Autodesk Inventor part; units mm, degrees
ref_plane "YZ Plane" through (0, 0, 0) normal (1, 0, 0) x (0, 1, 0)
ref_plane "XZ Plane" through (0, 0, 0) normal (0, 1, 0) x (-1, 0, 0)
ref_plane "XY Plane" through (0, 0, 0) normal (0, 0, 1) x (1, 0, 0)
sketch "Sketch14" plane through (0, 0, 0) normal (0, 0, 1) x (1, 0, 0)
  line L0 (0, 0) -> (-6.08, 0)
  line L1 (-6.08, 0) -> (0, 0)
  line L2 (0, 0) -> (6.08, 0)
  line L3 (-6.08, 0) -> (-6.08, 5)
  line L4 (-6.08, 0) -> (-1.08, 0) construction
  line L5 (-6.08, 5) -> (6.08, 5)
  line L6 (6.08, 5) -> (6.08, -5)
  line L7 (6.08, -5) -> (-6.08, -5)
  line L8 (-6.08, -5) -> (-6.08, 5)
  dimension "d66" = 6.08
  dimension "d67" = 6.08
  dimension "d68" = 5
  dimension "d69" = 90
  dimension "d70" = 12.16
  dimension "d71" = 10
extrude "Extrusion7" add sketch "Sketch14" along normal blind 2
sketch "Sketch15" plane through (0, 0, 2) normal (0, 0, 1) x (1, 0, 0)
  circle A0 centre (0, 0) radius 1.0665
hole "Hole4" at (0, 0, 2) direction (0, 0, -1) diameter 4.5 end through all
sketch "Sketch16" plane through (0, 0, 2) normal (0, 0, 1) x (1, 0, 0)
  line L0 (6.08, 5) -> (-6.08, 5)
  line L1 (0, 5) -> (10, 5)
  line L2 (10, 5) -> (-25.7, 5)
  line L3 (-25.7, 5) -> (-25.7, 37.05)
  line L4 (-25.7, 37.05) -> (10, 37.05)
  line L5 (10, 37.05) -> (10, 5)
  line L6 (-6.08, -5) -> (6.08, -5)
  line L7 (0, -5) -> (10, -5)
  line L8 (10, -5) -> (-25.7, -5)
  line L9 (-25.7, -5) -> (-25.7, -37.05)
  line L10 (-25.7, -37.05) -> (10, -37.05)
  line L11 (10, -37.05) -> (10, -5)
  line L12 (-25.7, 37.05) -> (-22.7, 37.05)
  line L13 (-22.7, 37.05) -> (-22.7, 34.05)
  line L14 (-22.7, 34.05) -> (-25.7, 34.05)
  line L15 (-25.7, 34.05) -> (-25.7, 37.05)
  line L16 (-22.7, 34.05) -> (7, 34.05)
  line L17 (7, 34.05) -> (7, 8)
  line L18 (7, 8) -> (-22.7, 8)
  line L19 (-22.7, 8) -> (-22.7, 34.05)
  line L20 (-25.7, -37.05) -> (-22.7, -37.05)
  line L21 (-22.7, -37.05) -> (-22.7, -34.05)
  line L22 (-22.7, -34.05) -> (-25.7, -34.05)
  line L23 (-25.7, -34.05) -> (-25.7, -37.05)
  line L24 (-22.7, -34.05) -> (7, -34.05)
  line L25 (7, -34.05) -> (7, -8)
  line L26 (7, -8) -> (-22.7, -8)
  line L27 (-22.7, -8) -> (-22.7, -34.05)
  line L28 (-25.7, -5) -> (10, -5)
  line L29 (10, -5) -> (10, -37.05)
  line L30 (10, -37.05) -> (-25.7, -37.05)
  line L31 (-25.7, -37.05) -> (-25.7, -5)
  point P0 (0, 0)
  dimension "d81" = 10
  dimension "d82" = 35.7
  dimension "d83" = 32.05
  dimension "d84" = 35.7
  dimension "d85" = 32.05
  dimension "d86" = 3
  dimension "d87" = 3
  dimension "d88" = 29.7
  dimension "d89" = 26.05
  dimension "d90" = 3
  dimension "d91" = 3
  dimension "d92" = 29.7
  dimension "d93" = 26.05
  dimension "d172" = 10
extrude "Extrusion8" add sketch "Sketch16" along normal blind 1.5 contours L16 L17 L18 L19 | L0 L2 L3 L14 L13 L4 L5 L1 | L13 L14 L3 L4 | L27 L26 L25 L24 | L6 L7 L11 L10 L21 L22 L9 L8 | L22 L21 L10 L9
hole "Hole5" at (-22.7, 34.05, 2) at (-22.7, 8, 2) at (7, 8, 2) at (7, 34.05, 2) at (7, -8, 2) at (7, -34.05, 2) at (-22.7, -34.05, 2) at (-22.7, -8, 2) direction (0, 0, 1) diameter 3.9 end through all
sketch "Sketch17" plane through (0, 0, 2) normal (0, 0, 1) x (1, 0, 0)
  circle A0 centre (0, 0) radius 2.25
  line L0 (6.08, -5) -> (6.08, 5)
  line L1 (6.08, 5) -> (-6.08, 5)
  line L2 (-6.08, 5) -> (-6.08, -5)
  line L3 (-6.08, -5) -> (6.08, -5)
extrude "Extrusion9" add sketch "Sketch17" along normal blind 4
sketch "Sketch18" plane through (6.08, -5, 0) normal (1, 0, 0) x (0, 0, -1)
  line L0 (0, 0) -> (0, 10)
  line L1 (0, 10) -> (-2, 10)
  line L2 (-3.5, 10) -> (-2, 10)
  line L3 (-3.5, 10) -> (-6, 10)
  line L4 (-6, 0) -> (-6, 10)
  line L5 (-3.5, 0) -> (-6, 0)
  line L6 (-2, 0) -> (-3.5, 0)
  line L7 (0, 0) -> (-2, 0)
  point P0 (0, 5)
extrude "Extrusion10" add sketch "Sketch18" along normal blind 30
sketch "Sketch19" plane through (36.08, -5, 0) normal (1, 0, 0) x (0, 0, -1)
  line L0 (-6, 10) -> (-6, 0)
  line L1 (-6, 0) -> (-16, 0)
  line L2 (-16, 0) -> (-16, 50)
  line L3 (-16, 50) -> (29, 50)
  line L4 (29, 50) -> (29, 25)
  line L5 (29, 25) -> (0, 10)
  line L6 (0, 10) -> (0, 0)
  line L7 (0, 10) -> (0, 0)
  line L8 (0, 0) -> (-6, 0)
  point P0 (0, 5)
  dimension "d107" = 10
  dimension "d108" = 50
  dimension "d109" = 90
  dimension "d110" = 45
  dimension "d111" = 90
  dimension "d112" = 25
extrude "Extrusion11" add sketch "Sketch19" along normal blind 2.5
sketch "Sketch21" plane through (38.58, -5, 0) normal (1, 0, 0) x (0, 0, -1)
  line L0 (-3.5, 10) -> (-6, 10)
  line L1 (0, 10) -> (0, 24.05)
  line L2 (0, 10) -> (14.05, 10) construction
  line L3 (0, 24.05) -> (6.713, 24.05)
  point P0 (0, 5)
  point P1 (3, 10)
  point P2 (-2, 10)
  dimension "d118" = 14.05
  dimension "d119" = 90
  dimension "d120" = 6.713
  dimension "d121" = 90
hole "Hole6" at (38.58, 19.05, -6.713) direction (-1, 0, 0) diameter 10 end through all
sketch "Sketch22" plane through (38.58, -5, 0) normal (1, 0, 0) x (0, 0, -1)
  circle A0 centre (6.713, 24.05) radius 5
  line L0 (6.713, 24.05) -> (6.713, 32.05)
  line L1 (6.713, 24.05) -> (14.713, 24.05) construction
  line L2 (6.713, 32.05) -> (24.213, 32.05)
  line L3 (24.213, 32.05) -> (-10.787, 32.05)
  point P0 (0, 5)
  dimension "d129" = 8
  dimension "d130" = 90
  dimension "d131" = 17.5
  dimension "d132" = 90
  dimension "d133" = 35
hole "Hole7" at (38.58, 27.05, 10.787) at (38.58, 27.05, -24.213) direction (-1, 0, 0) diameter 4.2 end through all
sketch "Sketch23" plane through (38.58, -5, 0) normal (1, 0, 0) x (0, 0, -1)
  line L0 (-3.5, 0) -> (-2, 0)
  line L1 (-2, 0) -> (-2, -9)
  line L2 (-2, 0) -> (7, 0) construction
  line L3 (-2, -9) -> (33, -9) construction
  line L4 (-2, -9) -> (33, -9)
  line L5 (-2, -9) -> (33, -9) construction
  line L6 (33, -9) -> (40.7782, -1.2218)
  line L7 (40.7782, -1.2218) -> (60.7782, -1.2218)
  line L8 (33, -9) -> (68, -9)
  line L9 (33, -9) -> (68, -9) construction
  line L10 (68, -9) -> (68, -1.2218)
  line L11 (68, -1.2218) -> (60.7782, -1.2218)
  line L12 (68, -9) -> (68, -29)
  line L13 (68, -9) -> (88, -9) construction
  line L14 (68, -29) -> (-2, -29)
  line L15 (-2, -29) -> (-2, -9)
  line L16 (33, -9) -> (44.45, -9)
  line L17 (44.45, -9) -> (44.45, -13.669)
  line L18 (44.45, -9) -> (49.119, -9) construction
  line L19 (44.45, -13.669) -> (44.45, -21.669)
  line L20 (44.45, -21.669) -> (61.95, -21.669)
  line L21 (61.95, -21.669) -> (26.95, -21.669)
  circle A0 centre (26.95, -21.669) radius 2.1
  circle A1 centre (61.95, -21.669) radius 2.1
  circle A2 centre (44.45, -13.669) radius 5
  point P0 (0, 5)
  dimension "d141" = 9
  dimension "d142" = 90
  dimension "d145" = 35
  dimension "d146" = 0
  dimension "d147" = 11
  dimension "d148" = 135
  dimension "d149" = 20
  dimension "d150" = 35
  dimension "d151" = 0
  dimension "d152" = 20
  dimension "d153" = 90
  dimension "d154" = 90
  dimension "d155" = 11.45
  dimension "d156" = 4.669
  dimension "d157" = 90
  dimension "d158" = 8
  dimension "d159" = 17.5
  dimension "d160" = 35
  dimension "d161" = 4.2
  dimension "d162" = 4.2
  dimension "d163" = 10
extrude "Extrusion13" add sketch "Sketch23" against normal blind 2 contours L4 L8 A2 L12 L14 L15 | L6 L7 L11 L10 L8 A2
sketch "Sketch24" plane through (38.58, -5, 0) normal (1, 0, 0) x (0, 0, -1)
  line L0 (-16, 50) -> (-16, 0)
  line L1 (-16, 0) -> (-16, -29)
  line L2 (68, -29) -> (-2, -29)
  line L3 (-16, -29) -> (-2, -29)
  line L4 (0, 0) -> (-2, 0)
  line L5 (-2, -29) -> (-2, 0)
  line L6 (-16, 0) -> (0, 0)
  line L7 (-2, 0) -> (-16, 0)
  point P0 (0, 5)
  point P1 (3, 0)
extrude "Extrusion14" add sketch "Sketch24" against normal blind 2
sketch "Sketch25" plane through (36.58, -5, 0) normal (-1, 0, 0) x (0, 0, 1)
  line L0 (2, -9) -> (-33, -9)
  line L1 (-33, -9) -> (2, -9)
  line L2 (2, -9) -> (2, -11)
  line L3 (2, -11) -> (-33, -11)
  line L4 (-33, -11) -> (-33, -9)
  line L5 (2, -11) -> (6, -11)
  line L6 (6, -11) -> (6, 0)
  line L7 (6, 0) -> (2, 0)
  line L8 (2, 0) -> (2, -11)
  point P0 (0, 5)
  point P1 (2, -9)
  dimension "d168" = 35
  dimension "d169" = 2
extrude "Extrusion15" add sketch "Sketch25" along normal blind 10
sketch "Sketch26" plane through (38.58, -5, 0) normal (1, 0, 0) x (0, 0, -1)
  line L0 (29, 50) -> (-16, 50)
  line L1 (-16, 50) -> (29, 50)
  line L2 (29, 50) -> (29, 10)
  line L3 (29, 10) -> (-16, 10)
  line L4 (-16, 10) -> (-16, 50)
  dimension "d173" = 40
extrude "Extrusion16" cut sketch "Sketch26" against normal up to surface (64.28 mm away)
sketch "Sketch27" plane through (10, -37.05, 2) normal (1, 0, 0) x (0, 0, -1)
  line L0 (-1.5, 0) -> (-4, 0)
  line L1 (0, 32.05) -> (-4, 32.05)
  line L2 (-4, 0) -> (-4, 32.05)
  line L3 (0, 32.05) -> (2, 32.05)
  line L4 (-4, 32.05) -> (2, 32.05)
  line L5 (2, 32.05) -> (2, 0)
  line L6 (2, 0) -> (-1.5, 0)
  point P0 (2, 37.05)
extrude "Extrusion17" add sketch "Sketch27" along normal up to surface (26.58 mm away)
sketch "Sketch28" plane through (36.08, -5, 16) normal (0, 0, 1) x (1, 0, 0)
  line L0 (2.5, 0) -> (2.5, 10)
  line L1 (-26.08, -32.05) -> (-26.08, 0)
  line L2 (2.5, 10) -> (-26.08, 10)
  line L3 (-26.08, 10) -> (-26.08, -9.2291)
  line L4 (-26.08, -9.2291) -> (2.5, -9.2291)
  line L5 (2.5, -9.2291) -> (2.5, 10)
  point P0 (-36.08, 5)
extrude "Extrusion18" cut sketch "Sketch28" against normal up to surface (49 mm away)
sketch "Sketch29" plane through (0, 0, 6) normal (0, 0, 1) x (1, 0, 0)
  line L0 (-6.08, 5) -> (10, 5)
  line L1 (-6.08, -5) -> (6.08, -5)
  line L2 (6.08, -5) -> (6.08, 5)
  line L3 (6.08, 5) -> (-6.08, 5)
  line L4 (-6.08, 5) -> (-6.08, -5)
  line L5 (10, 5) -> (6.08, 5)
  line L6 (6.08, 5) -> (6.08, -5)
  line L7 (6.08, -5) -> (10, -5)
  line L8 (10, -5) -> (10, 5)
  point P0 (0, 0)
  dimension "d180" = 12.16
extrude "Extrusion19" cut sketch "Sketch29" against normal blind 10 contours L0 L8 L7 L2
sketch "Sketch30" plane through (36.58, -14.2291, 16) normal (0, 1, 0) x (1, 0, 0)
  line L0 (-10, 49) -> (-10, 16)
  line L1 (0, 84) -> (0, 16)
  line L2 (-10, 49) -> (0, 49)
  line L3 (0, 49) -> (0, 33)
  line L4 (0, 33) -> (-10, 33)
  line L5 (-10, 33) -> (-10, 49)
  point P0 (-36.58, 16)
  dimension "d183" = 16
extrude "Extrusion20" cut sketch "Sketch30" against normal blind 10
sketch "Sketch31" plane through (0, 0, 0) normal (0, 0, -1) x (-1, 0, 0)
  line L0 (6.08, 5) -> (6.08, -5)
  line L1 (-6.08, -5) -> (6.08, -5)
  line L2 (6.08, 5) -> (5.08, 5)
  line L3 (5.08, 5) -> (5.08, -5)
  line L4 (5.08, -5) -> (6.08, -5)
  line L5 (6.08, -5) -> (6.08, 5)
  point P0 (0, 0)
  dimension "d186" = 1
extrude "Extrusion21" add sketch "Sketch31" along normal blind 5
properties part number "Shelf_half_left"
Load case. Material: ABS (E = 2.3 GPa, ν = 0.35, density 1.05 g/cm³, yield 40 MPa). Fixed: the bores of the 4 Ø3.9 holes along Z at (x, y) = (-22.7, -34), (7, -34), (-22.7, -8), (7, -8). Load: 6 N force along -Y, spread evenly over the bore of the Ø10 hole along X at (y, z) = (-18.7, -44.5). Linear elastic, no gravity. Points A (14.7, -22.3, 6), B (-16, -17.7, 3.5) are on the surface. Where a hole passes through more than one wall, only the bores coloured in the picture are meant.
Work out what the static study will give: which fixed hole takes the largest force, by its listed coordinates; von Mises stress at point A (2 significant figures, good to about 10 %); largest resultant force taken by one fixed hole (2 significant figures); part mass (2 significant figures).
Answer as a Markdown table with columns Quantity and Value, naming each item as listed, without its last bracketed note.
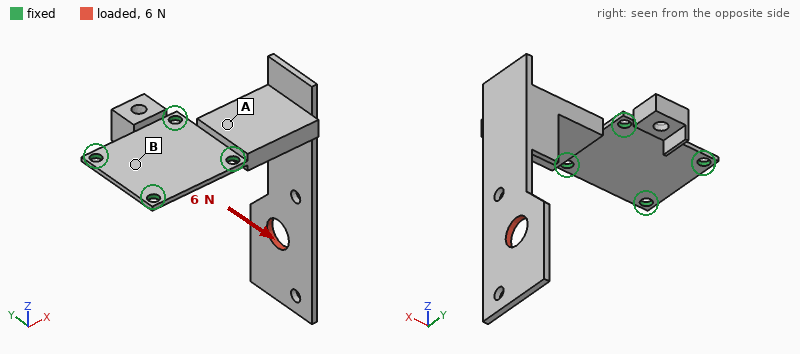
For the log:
| Quantity | Value |
|---|---|
| which fixed hole takes the largest force, by its listed coordinates | (7, -34) |
| von Mises stress at point A | 2.4 MPa |
| largest resultant force taken by one fixed hole | 14 N |
| part mass | 10 g |
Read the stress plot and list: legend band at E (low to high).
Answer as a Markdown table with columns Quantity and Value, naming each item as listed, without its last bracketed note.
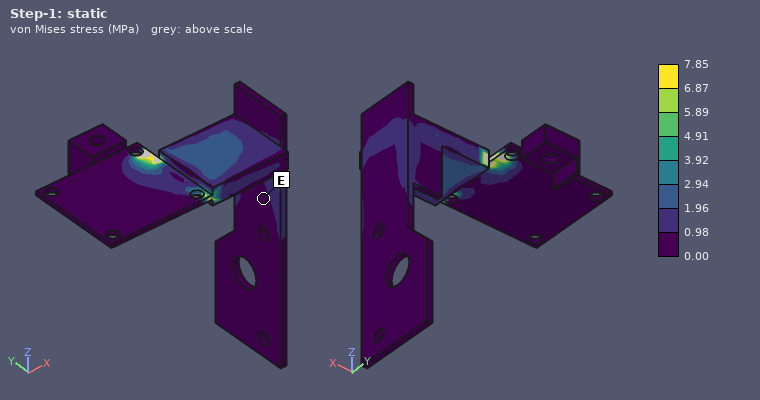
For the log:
| Quantity | Value |
|---|---|
| legend band at E | 0.00 to 0.98 MPa |
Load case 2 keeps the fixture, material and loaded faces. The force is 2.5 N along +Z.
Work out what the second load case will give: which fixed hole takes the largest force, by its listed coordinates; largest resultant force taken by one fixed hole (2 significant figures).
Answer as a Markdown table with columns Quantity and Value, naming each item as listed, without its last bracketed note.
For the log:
| Quantity | Value |
|---|---|
| which fixed hole takes the largest force, by its listed coordinates | (7, -8) |
| largest resultant force taken by one fixed hole | 1.9 N |
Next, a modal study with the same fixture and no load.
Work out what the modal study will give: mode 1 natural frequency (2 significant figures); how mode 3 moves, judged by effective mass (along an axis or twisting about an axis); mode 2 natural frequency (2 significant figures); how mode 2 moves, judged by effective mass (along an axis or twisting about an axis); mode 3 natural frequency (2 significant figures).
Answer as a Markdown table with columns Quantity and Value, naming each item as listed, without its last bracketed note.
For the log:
| Quantity | Value |
|---|---|
| mode 1 natural frequency | 85 Hz |
| how mode 3 moves, judged by effective mass | along Y |
| mode 2 natural frequency | 220 Hz |
| how mode 2 moves, judged by effective mass | along Z |
| mode 3 natural frequency | 300 Hz |
